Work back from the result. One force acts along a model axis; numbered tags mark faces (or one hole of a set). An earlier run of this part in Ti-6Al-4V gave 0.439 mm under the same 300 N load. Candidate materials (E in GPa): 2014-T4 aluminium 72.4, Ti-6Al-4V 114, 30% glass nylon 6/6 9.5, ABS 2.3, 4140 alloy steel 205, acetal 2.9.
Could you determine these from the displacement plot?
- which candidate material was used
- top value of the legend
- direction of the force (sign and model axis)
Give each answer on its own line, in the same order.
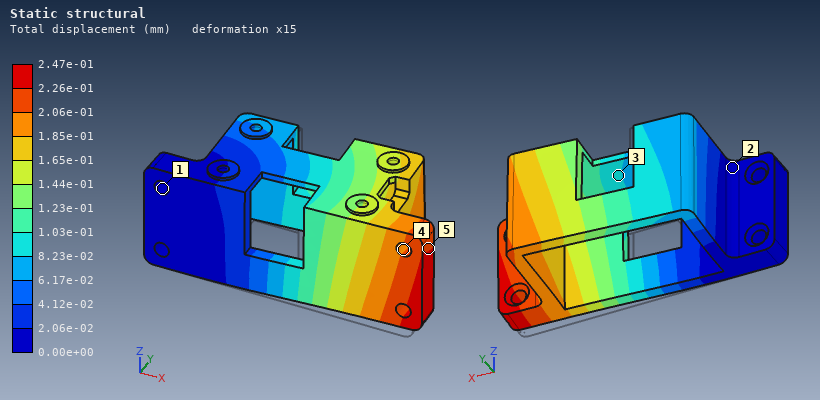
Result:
4140 alloy steel
2.47e-01 mm
+Y
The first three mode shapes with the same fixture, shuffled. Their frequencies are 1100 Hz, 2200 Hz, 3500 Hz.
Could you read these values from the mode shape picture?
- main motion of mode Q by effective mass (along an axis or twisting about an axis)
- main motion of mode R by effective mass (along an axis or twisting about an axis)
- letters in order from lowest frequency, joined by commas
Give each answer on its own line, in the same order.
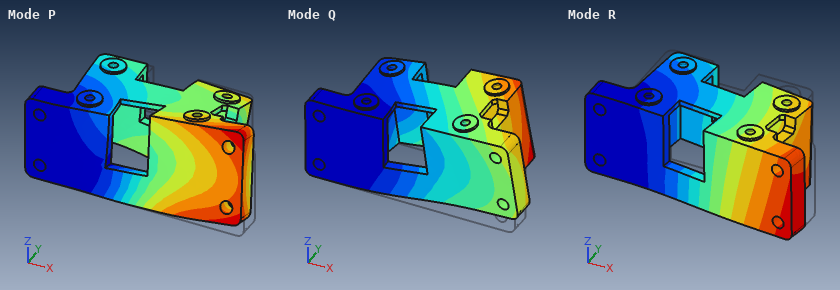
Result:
along Z
along Y
R, Q, P
